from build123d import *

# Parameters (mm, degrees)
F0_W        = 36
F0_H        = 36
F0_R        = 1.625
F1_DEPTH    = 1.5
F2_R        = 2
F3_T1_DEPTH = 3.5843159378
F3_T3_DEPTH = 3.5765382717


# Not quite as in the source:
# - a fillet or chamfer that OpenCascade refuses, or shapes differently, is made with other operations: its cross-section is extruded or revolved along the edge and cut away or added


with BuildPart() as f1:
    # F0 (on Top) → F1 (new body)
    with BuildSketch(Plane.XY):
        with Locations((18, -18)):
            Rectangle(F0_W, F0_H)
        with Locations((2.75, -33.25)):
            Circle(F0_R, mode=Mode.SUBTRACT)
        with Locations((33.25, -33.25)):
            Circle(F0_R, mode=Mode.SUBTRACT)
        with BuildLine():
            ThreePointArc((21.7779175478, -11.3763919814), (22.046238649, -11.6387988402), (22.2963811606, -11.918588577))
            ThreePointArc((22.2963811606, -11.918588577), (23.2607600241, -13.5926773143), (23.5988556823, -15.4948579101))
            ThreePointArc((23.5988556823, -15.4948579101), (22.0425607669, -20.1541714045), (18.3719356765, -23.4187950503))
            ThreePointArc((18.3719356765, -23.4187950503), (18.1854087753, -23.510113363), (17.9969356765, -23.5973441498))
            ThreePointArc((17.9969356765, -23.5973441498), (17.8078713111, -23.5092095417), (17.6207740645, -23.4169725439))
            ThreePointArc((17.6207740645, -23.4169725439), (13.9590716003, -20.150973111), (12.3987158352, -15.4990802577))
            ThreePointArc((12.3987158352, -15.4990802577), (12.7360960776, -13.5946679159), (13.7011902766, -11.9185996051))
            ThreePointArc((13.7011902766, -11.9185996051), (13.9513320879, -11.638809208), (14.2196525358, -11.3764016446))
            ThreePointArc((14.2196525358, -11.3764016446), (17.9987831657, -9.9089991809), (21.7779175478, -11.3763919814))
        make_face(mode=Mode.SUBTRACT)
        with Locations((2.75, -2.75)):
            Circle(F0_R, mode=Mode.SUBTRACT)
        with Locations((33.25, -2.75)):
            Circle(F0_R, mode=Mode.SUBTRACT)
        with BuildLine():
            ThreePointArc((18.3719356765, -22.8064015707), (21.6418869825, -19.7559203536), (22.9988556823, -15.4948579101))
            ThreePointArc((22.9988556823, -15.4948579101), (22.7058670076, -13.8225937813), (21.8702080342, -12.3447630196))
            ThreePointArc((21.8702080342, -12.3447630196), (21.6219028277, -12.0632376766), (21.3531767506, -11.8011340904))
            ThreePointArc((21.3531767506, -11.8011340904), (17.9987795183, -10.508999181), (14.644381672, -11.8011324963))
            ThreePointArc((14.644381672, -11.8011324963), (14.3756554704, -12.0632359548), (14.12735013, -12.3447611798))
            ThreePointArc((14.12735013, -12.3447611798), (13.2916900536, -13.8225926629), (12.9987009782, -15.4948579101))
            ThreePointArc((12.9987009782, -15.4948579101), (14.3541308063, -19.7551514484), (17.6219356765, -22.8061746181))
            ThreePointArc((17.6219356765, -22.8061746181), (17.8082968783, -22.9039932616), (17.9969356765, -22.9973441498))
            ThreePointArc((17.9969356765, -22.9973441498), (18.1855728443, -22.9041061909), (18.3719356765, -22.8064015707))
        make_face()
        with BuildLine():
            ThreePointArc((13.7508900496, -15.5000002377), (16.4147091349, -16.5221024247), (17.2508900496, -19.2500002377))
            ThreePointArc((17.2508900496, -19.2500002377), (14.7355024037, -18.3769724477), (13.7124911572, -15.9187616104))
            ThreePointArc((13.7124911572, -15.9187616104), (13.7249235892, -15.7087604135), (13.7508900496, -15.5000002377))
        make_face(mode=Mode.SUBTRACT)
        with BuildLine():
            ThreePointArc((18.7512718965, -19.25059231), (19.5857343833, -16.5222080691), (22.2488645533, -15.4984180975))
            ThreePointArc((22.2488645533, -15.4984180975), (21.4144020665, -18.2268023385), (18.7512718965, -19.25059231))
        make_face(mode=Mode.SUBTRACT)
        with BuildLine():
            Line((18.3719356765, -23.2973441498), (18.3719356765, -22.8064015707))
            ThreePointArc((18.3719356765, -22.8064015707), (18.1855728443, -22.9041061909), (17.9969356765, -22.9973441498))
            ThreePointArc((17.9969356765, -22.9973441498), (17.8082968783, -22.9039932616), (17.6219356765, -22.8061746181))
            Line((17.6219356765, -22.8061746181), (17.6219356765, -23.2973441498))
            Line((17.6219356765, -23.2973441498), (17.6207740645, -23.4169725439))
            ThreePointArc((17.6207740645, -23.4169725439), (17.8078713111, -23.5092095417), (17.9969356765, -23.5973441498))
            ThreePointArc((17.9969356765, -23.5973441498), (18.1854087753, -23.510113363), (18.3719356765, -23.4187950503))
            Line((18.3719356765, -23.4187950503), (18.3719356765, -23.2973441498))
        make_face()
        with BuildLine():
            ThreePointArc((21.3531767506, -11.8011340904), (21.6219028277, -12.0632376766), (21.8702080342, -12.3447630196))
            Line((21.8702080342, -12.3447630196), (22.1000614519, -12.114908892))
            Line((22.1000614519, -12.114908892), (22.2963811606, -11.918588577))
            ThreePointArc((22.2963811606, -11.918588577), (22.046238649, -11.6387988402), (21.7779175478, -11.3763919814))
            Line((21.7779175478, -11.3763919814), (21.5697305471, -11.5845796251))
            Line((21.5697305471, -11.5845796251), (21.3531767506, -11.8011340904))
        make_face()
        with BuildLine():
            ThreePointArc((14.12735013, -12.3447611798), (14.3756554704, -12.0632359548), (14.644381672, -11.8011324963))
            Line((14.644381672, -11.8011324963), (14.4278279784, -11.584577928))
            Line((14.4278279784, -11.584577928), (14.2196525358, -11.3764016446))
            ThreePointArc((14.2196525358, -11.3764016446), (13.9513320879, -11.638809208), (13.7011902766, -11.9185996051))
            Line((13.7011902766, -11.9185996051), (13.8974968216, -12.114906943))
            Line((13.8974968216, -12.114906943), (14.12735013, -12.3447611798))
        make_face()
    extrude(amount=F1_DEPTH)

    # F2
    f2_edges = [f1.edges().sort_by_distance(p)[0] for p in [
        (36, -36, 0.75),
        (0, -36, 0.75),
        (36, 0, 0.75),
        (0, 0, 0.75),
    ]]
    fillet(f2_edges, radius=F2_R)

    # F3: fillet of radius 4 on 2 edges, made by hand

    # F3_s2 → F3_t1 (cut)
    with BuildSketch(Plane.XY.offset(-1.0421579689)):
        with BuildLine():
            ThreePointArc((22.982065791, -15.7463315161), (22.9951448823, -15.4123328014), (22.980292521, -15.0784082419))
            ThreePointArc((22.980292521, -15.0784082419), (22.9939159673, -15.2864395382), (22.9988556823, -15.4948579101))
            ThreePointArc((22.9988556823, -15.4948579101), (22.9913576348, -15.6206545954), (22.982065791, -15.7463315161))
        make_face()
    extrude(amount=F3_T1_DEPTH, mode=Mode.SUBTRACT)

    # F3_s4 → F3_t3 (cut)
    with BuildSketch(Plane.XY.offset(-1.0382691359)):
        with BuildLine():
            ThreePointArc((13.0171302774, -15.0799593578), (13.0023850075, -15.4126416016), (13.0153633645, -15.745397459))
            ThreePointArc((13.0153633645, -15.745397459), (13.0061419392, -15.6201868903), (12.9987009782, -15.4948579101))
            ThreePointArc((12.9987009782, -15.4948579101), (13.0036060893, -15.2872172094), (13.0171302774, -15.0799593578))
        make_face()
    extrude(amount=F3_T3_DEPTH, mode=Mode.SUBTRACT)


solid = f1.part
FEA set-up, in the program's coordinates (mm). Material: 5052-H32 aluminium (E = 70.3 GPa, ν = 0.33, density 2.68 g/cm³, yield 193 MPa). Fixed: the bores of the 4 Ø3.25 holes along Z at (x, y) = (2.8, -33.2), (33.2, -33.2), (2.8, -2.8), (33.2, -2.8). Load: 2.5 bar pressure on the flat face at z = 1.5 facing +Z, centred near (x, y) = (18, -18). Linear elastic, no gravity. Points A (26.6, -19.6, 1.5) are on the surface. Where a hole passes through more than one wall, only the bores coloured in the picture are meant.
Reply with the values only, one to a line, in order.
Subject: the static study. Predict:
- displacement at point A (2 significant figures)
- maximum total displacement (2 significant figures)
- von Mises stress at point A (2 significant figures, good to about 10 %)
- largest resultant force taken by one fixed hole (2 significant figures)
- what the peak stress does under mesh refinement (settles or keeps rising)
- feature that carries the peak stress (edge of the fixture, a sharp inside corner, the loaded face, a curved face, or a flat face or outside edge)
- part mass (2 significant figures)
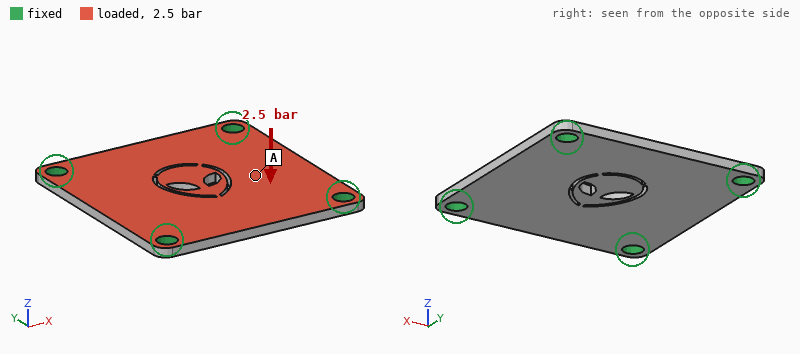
52 µm
75 µm
28 MPa
76 N
keeps rising
edge of the fixture
4.9 g
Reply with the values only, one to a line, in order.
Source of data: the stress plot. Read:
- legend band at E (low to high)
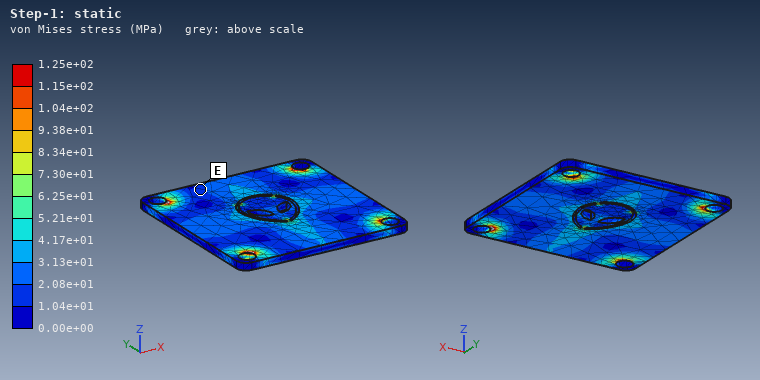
1.04e+01 to 2.08e+01 MPa
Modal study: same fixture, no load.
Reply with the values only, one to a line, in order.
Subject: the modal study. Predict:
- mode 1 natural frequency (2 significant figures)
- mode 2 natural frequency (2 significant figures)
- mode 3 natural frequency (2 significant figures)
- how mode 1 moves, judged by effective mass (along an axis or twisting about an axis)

5900 Hz
10 kHz
10 kHz
along Z
